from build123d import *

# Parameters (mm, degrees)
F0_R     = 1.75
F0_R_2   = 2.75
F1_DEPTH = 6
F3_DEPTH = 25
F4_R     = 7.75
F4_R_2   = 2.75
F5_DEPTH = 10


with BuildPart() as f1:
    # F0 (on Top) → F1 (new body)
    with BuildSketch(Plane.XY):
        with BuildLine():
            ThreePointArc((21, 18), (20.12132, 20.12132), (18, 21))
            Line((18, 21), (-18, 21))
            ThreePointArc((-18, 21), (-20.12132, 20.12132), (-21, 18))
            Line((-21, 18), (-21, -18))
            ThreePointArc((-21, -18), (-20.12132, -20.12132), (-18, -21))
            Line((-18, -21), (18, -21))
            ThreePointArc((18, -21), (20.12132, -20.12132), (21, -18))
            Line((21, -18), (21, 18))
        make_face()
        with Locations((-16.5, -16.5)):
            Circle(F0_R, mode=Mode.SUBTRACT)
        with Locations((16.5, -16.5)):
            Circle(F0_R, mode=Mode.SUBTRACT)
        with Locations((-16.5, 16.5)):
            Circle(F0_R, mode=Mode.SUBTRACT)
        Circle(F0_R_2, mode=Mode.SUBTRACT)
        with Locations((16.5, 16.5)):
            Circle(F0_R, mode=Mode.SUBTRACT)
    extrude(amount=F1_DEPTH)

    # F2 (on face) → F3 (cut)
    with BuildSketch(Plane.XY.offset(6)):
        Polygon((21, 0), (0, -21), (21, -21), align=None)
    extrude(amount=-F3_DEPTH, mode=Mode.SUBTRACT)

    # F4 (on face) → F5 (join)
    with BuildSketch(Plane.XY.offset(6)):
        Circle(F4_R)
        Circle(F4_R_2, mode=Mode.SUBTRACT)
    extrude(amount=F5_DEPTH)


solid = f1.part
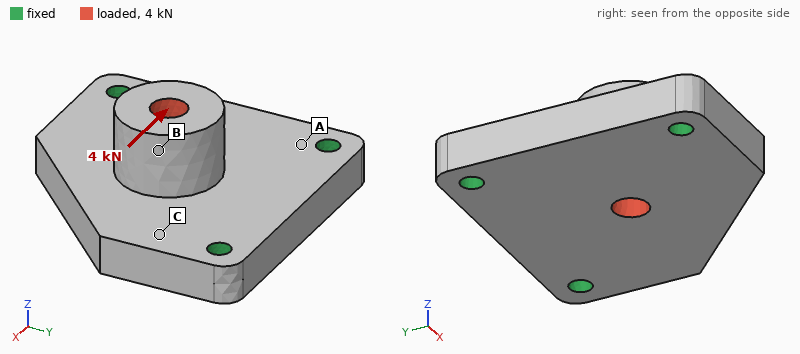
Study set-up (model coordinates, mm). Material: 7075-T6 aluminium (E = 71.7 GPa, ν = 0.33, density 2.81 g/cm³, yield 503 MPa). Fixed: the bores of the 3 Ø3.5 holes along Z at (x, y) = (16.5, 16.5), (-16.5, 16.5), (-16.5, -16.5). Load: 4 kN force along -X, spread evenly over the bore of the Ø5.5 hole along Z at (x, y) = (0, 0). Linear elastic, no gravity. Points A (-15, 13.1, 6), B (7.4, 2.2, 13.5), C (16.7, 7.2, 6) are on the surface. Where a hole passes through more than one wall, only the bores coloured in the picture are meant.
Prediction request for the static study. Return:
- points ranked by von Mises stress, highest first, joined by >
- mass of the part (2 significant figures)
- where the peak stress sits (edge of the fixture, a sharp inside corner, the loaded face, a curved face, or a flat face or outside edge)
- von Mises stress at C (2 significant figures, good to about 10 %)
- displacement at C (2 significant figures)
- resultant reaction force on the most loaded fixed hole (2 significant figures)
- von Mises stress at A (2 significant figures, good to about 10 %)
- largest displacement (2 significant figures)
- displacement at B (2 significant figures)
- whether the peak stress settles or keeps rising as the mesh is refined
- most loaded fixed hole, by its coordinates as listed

A > C > B
30 g
edge of the fixture
22 MPa
13 µm
1.7 kN
32 MPa
41 µm
35 µm
keeps rising
(-16.5, 16.5)
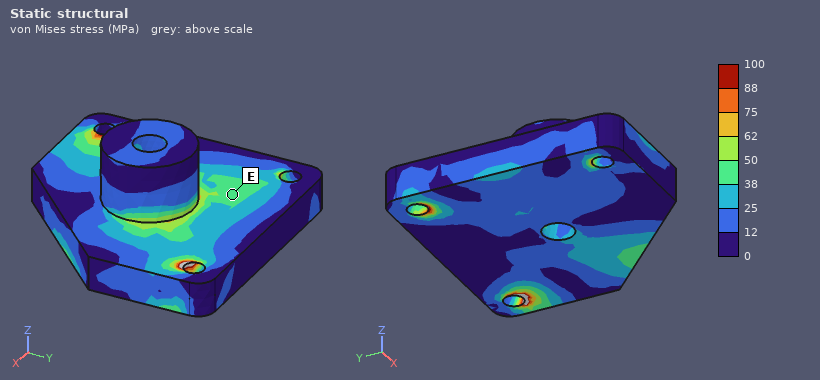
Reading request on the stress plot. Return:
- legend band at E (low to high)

38 to 50 MPa
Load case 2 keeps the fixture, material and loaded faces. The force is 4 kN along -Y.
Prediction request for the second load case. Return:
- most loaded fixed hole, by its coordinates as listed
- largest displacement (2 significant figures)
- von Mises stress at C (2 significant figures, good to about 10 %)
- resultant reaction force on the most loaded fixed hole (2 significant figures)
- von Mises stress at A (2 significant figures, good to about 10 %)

(-16.5, 16.5)
41 µm
34 MPa
1.7 kN
36 MPa
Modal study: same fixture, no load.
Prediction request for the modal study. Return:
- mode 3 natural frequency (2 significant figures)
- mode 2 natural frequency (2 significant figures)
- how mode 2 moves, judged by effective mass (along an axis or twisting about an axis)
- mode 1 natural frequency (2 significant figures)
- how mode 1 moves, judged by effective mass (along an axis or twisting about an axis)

21 kHz
18 kHz
along Z
9300 Hz
along Z
